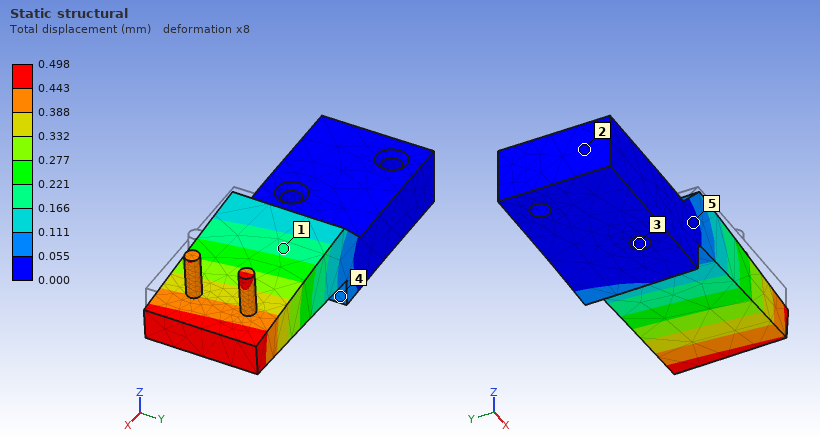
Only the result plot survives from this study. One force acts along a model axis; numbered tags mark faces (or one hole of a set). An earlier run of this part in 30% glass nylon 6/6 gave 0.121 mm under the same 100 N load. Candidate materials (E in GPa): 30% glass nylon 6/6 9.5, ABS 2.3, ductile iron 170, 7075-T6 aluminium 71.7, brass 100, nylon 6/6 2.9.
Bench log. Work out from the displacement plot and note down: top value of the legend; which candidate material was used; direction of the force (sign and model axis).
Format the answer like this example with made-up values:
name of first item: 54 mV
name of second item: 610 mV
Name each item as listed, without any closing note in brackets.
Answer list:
top value of the legend: 0.498 mm
which candidate material was used: ABS
direction of the force: -Z
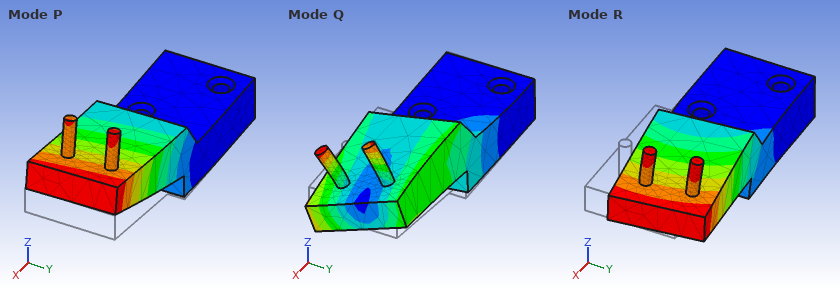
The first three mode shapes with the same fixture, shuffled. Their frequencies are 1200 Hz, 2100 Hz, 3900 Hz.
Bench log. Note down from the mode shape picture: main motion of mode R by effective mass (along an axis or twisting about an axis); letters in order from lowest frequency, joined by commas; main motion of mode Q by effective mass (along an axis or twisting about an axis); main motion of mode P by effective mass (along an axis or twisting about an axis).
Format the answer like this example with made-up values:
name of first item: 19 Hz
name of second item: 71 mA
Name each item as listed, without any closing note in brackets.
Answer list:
main motion of mode R by effective mass: along Y
letters in order from lowest frequency, joined by commas: P, R, Q
main motion of mode Q by effective mass: twisting about X
main motion of mode P by effective mass: along Z
